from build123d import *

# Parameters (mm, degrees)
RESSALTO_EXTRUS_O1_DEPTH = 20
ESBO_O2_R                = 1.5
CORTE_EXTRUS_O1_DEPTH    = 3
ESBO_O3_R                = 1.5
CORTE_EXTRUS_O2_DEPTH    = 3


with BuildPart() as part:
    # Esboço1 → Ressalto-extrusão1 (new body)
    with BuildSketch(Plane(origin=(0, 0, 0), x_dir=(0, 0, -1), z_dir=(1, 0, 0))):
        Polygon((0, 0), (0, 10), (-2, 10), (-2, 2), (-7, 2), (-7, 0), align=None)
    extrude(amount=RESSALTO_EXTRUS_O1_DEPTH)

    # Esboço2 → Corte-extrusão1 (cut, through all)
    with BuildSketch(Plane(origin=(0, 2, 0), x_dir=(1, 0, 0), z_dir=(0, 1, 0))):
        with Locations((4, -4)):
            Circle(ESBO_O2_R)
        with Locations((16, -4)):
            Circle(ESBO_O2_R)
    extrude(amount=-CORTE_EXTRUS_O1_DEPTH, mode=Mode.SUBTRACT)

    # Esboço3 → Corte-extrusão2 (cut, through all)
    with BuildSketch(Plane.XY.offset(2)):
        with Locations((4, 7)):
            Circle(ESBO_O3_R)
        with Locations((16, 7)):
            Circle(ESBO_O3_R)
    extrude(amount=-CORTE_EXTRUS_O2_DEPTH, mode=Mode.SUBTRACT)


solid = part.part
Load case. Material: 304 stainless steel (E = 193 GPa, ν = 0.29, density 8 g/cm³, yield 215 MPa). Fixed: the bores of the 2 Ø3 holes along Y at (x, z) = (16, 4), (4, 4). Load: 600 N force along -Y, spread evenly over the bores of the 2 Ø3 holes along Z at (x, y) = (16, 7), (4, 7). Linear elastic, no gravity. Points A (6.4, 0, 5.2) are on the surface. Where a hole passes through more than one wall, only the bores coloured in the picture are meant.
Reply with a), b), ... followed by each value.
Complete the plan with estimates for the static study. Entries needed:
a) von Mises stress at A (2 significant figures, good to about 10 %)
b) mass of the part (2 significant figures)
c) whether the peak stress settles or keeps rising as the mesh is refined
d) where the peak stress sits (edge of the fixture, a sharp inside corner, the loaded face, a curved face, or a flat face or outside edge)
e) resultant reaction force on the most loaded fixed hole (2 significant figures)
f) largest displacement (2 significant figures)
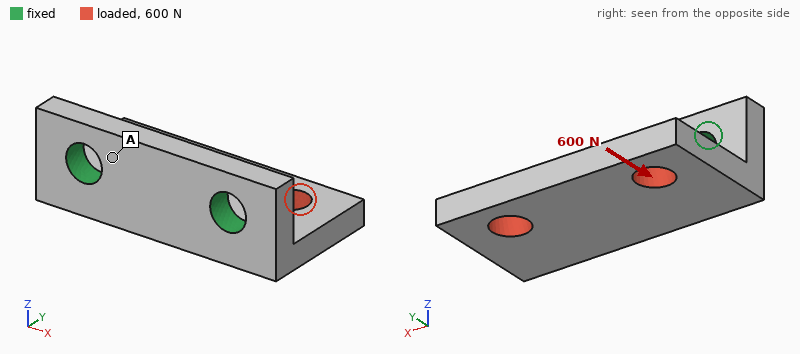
a) 19 MPa
b) 4.3 g
c) keeps rising
d) edge of the fixture
e) 300 N
f) 7.5 µm
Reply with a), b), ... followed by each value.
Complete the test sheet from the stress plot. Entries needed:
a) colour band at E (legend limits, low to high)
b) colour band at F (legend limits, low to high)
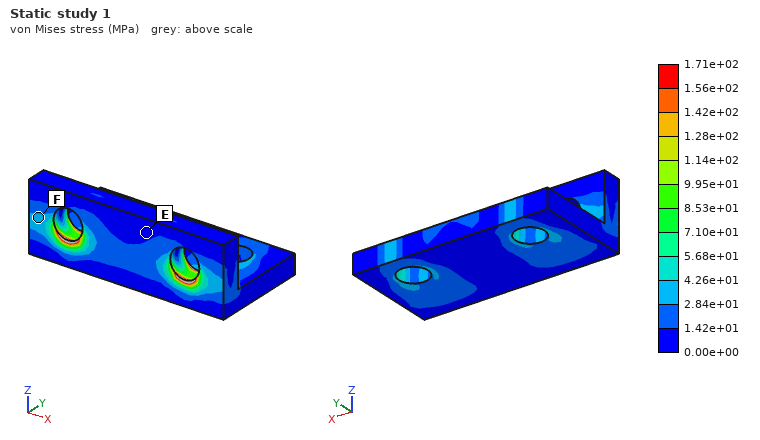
a) 0.00e+00 to 1.42e+01 MPa
b) 2.84e+01 to 4.26e+01 MPa
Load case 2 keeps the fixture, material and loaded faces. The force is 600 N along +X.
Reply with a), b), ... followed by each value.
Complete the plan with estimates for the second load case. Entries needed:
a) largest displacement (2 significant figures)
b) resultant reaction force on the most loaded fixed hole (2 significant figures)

a) 6.3 µm
b) 410 N
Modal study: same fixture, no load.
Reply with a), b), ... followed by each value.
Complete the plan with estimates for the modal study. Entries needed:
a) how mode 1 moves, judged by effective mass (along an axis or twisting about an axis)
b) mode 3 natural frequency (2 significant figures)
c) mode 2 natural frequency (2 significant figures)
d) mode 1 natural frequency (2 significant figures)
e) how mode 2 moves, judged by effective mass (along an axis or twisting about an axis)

a) along Z
b) 41 kHz
c) 23 kHz
d) 15 kHz
e) twisting about Y
